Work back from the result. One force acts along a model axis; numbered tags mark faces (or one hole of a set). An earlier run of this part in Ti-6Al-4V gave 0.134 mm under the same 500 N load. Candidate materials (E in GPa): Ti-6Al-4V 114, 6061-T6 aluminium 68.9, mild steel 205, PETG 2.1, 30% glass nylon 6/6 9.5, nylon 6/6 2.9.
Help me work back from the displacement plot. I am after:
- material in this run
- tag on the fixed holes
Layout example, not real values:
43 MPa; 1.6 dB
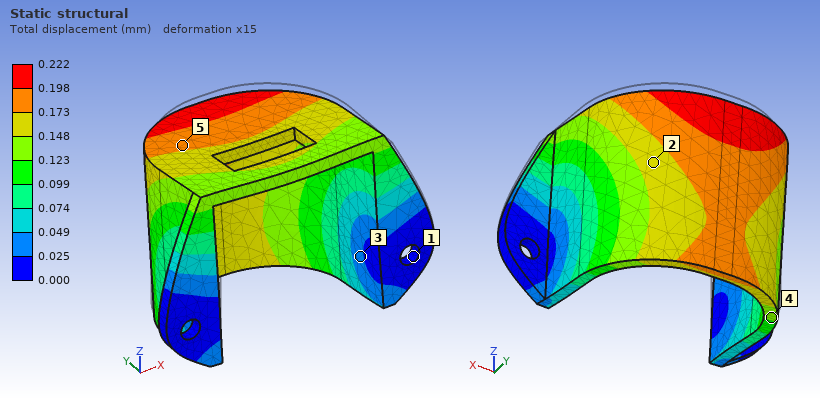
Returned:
6061-T6 aluminium; 1
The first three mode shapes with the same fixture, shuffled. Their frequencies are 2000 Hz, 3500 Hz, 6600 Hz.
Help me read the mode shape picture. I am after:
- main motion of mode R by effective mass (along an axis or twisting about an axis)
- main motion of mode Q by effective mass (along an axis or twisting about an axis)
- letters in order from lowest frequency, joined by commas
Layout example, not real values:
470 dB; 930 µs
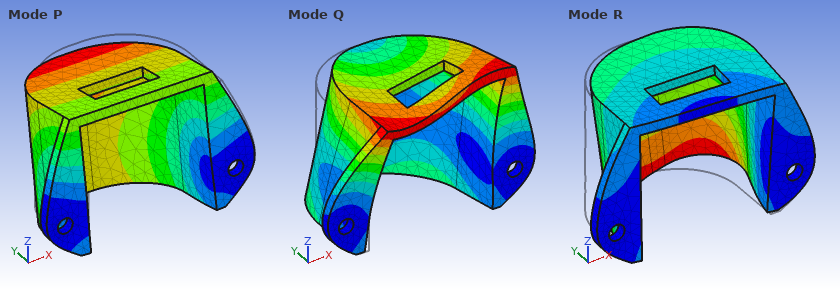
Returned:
along X; along X; P, R, Q
